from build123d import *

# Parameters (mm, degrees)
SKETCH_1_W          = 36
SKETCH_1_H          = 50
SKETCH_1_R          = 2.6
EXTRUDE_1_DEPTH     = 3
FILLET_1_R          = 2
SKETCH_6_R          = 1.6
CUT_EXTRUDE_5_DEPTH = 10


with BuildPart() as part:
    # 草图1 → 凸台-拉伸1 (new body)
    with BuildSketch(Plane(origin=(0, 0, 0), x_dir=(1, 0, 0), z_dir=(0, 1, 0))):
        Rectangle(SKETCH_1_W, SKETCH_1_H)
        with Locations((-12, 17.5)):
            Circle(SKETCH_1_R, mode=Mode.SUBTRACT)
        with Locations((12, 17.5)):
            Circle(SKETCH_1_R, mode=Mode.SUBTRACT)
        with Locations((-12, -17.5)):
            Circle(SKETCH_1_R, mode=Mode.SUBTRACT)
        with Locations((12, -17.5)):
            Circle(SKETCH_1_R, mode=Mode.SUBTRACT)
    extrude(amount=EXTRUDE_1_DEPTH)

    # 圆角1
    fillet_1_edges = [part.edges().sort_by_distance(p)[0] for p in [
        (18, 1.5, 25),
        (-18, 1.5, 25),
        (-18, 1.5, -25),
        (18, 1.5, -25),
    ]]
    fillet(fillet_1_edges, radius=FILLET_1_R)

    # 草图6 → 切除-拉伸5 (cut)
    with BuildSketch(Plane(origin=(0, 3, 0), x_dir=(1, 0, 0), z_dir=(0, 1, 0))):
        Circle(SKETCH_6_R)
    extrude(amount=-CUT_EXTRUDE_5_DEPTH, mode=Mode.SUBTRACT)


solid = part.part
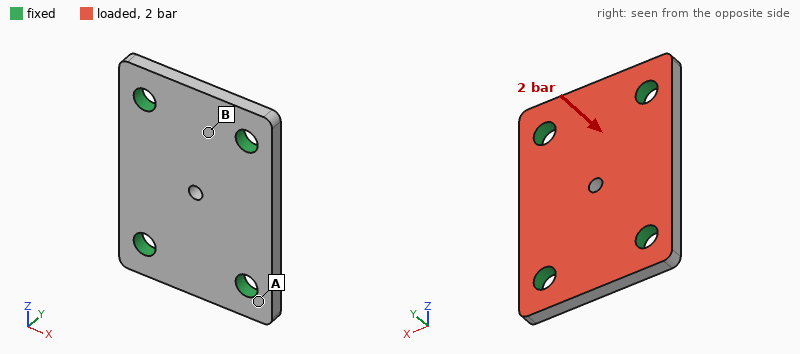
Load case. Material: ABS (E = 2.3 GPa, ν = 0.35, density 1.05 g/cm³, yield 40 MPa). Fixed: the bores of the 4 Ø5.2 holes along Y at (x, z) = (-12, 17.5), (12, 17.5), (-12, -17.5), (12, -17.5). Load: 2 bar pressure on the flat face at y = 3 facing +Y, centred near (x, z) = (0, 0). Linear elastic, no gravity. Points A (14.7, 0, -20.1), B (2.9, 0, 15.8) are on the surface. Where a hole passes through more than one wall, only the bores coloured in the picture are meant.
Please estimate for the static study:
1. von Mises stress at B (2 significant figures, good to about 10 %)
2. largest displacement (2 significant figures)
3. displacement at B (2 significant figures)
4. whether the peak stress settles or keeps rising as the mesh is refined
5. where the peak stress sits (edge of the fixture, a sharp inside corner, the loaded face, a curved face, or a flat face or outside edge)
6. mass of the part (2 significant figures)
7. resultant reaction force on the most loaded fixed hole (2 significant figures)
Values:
3.9 MPa
0.15 mm
0.037 mm
keeps rising
edge of the fixture
5.4 g
85 N
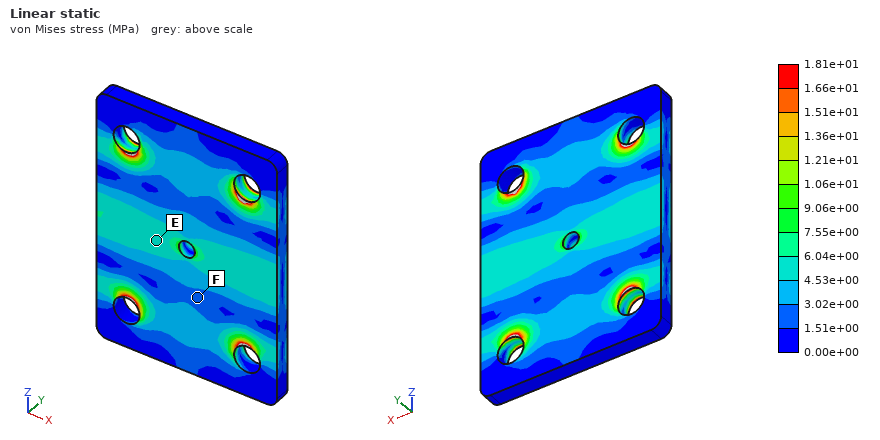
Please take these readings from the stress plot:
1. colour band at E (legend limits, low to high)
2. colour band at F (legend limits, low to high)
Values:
4.53e+00 to 6.04e+00 MPa
1.51e+00 to 3.02e+00 MPa
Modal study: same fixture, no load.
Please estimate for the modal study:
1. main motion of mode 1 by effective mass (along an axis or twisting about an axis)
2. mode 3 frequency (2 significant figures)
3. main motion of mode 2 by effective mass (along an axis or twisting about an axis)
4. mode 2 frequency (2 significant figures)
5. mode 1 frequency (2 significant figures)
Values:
along Y
6400 Hz
twisting about Z
4900 Hz
3900 Hz
